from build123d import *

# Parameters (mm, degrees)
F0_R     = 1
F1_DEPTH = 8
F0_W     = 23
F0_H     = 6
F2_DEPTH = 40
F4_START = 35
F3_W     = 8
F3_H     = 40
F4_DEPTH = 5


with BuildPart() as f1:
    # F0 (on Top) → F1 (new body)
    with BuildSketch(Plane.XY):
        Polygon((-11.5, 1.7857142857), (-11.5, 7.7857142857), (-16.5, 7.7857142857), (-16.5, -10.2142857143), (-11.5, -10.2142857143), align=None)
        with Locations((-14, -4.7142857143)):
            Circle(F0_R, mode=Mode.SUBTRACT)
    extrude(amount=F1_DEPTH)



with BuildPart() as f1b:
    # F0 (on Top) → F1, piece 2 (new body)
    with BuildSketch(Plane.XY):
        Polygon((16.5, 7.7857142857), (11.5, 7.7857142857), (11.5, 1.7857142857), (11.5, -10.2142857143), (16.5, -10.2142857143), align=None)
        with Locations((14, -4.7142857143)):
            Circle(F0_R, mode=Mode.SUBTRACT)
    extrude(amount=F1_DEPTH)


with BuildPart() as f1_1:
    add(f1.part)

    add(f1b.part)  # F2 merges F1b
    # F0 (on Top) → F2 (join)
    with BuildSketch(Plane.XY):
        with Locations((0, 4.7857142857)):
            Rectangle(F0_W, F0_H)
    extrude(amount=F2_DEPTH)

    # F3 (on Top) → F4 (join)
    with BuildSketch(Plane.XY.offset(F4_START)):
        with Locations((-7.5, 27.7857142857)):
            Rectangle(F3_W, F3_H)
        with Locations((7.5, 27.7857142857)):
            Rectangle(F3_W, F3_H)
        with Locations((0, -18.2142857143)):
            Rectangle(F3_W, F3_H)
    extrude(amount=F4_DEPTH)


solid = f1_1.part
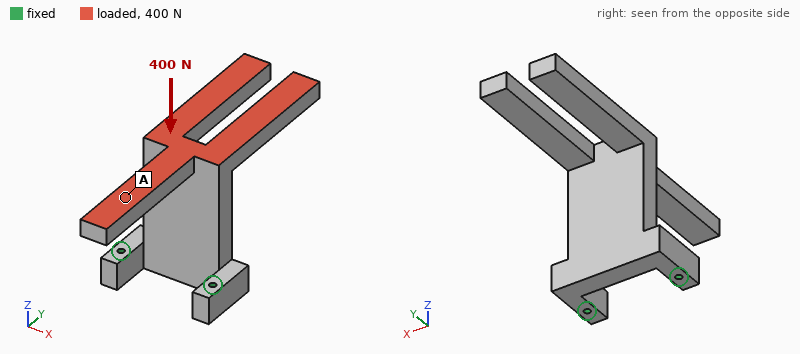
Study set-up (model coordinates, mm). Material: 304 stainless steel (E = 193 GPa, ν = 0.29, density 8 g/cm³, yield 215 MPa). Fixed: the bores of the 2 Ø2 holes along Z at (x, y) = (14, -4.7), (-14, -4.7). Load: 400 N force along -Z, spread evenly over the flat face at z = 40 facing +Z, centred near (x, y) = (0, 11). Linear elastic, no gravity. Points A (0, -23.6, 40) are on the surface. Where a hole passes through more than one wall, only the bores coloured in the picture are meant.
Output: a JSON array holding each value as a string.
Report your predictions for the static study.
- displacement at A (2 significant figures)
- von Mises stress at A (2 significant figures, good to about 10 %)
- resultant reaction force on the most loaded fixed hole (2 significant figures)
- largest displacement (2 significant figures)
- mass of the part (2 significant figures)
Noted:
["0.040 mm", "9.6 MPa", "200 N", "0.16 mm", "94 g"]
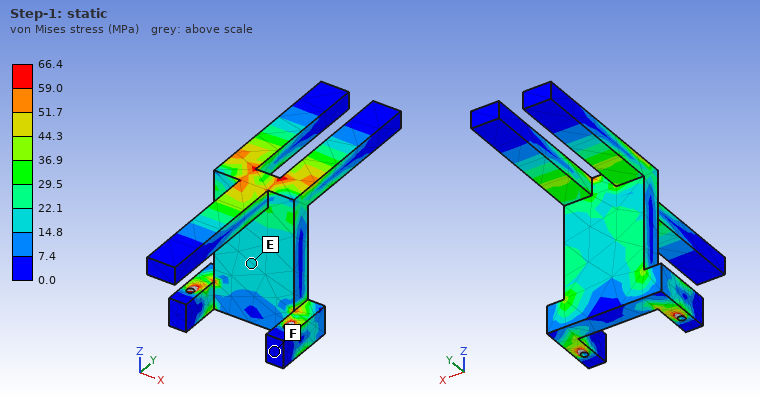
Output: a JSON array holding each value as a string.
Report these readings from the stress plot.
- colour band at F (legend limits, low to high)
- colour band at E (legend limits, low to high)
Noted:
["0.0 to 7.4 MPa", "14.8 to 22.1 MPa"]
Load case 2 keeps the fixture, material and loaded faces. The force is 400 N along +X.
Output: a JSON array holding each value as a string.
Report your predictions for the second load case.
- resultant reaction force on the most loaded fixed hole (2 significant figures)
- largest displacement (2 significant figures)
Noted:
["570 N", "73 µm"]
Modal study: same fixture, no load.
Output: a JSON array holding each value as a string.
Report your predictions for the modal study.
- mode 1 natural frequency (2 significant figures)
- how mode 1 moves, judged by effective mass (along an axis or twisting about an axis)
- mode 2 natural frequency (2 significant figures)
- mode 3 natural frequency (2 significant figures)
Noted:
["880 Hz", "along Y", "1600 Hz", "2100 Hz"]
